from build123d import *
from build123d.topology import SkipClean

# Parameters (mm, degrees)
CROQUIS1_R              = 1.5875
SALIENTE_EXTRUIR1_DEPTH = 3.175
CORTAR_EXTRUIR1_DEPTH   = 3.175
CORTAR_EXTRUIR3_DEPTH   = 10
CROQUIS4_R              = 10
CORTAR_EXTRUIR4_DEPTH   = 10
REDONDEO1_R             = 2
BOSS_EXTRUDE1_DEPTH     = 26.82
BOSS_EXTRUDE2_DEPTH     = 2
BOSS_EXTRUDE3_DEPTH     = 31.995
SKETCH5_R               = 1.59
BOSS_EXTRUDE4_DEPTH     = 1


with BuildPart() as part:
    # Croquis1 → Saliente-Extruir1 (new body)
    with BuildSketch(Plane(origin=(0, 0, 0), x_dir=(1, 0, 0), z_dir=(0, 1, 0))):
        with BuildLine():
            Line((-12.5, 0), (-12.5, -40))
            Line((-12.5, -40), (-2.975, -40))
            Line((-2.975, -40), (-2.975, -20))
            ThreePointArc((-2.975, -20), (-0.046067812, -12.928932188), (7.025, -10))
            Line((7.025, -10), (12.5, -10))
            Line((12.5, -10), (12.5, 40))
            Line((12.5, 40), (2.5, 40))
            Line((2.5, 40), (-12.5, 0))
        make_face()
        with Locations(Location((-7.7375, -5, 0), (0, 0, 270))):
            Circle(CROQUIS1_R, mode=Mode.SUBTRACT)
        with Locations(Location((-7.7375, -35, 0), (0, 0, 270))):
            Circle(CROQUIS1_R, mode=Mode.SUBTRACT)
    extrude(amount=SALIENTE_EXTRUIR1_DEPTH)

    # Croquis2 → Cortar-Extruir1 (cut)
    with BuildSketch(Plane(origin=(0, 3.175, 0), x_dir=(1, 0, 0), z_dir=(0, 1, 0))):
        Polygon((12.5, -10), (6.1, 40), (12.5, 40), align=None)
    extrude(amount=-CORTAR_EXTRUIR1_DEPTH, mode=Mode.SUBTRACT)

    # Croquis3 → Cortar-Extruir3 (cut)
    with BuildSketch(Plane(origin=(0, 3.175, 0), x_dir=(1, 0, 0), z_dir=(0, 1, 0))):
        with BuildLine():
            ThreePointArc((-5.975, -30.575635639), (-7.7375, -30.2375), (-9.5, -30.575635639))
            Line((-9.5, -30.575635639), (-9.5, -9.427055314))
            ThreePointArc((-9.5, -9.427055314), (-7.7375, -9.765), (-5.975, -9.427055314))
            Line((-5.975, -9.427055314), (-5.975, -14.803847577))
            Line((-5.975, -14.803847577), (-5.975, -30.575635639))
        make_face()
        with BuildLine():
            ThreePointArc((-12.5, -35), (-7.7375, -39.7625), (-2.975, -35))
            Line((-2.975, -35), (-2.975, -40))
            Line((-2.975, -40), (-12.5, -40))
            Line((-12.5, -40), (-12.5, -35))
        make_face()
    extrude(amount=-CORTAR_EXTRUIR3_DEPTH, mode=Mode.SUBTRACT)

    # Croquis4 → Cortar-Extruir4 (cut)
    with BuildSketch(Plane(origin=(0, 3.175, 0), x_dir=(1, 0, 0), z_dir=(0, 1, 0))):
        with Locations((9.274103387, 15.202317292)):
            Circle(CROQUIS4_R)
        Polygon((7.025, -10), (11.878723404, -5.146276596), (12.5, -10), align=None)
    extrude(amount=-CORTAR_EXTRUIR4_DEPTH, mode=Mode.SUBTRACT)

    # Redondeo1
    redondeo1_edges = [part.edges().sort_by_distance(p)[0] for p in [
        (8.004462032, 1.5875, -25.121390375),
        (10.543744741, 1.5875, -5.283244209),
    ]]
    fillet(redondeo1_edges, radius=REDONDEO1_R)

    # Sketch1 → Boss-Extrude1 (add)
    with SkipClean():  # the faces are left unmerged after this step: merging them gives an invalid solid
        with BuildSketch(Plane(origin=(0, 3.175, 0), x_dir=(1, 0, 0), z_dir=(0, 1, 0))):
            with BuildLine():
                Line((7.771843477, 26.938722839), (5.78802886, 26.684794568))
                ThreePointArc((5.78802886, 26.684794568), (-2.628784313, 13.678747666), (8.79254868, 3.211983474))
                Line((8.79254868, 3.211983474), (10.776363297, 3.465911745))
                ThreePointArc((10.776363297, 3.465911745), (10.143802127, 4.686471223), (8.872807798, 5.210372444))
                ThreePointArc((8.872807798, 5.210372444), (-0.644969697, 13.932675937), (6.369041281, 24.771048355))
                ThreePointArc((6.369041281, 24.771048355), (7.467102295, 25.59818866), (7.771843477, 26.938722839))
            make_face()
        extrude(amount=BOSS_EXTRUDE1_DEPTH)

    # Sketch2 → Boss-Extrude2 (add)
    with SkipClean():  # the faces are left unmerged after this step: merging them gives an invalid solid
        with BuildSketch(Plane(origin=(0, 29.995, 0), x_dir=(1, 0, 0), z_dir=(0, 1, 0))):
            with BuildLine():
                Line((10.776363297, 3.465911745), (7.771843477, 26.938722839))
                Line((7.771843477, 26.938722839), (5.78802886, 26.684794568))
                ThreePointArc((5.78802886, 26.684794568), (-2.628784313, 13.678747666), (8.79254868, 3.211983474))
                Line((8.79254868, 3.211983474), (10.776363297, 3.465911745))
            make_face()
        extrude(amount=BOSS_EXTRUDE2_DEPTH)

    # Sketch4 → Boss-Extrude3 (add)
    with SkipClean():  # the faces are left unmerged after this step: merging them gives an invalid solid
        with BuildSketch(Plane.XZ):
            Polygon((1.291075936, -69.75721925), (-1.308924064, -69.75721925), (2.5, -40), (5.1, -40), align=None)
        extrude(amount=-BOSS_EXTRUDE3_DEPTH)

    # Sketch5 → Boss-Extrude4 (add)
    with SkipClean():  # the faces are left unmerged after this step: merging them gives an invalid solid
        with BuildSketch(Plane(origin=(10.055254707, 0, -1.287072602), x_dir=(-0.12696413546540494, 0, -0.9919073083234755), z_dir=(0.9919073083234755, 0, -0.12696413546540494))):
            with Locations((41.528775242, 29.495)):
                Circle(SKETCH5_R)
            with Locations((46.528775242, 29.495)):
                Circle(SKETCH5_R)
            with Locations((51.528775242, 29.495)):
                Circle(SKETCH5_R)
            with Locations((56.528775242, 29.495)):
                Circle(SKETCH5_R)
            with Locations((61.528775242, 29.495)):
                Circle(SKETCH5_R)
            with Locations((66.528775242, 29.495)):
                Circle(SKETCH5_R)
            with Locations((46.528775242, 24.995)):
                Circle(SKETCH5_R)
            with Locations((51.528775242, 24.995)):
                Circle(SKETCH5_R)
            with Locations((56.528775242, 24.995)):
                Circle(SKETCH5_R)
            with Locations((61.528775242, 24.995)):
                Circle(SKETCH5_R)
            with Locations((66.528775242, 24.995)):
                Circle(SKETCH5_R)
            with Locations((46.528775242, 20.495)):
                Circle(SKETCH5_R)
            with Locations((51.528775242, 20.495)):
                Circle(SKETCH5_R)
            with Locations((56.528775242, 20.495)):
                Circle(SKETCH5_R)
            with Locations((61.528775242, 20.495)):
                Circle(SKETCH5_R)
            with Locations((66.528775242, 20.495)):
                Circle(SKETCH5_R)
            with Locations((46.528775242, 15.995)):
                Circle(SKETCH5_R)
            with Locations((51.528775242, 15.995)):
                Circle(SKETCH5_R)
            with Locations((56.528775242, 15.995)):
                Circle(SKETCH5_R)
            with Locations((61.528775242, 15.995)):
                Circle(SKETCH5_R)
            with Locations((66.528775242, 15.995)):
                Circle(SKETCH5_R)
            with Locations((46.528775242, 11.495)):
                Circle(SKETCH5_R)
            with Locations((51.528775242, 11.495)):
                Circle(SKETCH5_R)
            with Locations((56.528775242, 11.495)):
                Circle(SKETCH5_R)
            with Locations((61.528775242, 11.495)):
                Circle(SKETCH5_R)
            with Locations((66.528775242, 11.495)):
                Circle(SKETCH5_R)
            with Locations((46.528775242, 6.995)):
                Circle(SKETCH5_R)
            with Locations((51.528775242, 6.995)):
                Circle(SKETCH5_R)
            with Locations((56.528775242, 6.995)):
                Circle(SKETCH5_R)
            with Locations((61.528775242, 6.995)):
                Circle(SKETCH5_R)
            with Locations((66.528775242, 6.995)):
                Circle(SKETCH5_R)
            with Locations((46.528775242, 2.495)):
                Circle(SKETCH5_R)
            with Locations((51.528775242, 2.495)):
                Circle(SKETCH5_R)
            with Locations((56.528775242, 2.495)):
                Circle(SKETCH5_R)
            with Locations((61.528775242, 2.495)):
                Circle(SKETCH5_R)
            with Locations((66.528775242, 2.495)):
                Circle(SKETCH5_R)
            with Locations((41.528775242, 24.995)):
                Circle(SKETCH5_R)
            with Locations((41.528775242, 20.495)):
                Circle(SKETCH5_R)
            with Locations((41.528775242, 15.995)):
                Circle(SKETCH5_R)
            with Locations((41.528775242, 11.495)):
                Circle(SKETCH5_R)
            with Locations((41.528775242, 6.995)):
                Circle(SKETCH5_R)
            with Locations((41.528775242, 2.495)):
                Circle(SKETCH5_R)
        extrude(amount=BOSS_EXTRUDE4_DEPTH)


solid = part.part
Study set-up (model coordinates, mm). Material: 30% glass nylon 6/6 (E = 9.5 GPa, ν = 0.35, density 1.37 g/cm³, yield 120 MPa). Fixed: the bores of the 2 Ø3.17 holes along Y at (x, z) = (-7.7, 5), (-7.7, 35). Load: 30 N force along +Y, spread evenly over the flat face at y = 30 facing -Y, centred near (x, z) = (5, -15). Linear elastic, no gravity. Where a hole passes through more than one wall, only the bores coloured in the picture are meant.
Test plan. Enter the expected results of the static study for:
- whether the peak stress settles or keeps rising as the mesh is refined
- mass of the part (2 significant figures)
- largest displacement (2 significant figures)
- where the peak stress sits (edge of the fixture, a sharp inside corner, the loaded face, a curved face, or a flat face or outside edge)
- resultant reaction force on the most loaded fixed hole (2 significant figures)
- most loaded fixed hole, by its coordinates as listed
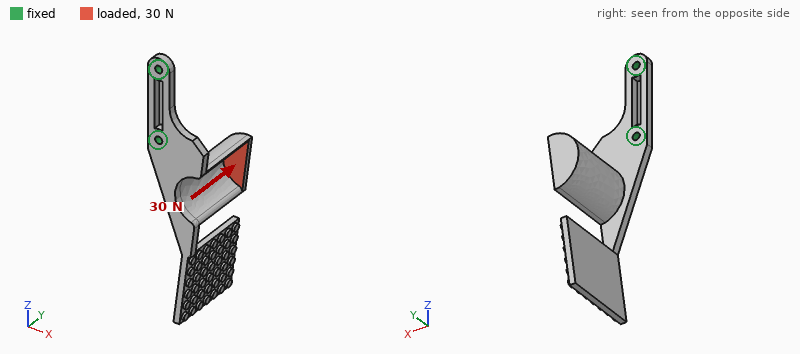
keeps rising
11 g
1.3 mm
edge of the fixture
34 N
(-7.7, 5)
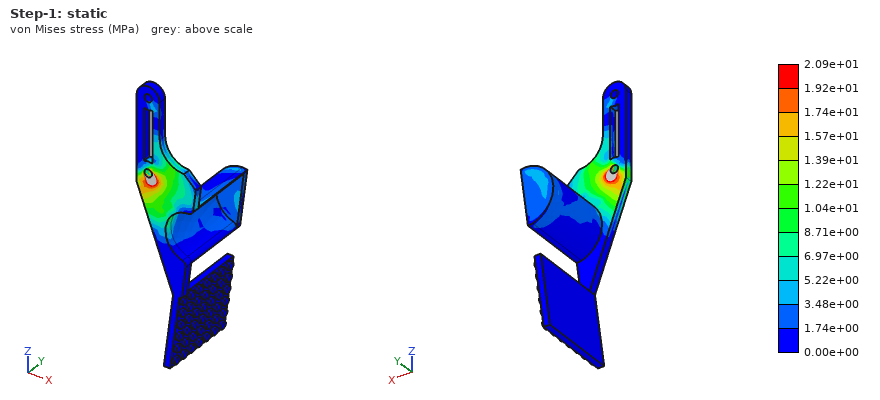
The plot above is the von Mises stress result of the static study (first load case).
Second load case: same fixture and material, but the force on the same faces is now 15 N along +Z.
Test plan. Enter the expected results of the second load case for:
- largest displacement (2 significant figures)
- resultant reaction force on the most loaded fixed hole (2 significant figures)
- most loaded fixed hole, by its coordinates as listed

1.2 mm
11 N
(-7.7, 5)
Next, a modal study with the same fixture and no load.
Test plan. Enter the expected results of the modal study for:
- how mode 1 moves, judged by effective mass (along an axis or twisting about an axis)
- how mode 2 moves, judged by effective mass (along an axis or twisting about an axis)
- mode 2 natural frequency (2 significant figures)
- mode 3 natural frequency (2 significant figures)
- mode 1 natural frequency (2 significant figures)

along Y
along X
230 Hz
530 Hz
160 Hz
